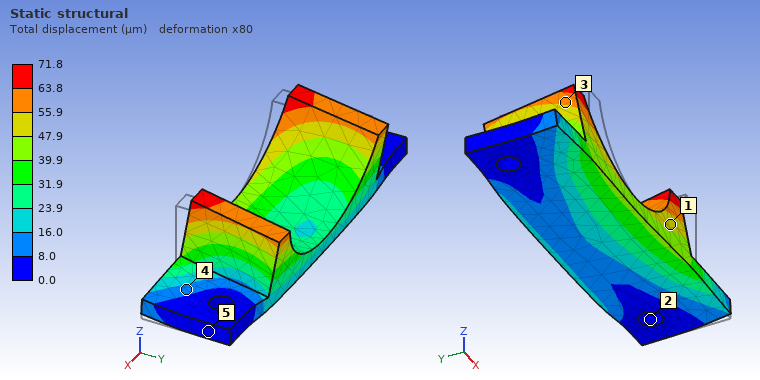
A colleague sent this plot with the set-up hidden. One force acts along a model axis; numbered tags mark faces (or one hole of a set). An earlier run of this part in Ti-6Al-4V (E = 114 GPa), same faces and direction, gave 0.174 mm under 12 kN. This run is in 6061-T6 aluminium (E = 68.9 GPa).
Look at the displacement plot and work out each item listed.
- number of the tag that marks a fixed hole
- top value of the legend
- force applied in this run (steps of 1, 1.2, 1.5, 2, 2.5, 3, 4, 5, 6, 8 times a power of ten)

2
71.8 µm
3 kN
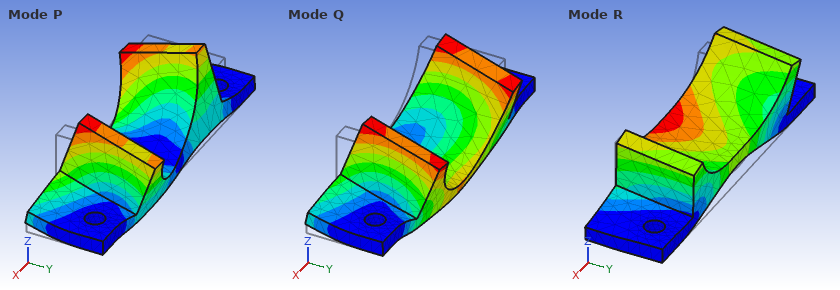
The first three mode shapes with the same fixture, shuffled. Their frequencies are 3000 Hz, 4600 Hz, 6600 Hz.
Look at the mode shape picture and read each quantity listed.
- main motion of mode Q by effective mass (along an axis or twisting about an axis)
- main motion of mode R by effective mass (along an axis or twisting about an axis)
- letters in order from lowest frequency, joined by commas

along Y
along Z
R, Q, P
